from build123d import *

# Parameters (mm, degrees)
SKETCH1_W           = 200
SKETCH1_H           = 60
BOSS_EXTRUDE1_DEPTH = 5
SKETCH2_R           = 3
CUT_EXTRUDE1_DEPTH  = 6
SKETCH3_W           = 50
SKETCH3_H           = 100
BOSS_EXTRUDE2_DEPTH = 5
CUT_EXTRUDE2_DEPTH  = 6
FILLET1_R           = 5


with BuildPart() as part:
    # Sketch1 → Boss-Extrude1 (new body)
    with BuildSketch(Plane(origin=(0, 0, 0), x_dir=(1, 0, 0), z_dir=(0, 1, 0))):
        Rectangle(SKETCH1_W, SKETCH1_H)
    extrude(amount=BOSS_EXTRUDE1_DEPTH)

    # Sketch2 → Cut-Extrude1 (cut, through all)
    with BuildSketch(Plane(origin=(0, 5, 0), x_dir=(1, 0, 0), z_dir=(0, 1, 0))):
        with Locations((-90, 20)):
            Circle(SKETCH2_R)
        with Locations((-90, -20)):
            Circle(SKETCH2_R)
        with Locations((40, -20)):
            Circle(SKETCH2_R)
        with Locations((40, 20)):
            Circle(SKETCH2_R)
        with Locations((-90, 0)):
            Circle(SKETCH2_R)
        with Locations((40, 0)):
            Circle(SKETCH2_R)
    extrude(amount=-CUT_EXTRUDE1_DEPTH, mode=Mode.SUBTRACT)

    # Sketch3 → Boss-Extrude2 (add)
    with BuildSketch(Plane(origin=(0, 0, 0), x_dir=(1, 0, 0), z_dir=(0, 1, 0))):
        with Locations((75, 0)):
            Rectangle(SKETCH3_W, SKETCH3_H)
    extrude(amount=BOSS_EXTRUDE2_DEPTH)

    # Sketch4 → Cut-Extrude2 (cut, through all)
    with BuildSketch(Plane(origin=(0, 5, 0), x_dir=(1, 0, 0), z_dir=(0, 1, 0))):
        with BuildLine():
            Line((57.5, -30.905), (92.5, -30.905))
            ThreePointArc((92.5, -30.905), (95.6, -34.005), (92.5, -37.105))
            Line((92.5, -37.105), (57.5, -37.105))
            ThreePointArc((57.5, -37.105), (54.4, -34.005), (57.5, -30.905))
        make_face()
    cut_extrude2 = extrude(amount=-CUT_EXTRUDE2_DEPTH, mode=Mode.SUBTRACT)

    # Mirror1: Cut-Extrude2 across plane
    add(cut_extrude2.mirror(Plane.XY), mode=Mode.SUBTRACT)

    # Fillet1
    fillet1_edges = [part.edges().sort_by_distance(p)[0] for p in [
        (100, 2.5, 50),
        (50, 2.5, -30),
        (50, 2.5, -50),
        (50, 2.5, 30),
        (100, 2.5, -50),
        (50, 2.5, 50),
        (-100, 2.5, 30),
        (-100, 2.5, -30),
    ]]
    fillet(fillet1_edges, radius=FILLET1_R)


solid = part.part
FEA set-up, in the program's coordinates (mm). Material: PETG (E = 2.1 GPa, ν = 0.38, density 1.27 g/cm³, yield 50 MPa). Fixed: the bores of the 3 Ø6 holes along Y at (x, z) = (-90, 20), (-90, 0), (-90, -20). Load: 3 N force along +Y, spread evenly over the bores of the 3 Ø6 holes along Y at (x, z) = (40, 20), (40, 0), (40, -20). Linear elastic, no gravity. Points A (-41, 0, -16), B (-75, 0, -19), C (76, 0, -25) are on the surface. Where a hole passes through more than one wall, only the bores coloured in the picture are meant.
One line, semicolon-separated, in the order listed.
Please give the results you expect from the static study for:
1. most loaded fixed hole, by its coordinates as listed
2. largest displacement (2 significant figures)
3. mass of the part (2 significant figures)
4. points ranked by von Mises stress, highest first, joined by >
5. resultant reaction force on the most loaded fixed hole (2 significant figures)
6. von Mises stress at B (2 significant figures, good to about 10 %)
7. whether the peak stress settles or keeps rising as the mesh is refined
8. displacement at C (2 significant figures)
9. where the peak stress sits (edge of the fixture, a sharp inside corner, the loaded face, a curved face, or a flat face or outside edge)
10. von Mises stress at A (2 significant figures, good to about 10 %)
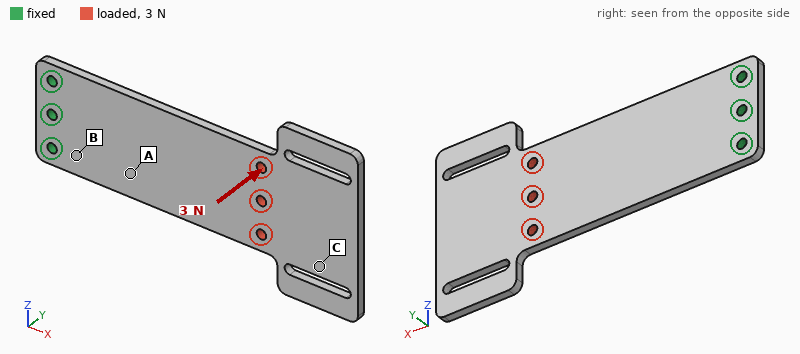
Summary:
(-90, 0); 2.7 mm; 85 g; B > A > C; 4.3 N; 1.3 MPa; keeps rising; 2.2 mm; edge of the fixture; 0.94 MPa
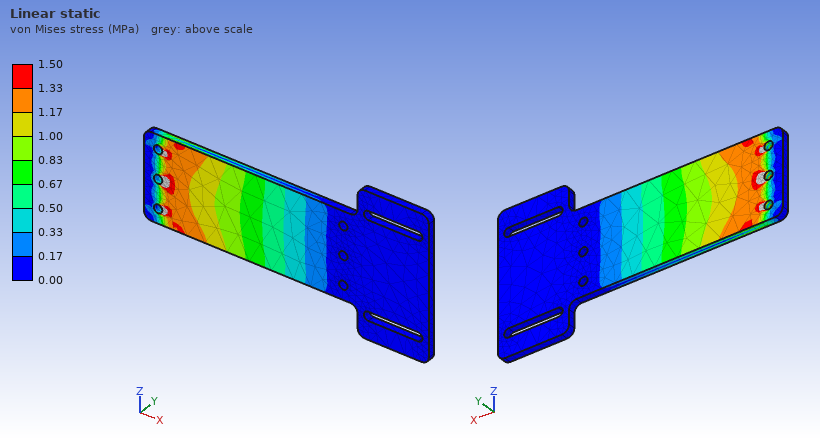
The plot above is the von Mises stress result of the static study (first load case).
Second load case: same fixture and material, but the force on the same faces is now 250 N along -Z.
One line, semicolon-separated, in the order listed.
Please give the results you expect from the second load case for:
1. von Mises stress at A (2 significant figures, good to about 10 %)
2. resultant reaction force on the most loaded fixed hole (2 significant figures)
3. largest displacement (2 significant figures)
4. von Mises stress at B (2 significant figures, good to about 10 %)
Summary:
3.9 MPa; 760 N; 2.0 mm; 7.1 MPa
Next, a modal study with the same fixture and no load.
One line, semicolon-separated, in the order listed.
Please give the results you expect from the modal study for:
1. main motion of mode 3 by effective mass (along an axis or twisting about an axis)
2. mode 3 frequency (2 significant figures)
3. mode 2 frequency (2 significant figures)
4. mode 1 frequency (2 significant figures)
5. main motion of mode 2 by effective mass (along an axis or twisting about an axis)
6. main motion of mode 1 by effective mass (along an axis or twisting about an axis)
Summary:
along Y; 170 Hz; 110 Hz; 26 Hz; twisting about X; along Y
